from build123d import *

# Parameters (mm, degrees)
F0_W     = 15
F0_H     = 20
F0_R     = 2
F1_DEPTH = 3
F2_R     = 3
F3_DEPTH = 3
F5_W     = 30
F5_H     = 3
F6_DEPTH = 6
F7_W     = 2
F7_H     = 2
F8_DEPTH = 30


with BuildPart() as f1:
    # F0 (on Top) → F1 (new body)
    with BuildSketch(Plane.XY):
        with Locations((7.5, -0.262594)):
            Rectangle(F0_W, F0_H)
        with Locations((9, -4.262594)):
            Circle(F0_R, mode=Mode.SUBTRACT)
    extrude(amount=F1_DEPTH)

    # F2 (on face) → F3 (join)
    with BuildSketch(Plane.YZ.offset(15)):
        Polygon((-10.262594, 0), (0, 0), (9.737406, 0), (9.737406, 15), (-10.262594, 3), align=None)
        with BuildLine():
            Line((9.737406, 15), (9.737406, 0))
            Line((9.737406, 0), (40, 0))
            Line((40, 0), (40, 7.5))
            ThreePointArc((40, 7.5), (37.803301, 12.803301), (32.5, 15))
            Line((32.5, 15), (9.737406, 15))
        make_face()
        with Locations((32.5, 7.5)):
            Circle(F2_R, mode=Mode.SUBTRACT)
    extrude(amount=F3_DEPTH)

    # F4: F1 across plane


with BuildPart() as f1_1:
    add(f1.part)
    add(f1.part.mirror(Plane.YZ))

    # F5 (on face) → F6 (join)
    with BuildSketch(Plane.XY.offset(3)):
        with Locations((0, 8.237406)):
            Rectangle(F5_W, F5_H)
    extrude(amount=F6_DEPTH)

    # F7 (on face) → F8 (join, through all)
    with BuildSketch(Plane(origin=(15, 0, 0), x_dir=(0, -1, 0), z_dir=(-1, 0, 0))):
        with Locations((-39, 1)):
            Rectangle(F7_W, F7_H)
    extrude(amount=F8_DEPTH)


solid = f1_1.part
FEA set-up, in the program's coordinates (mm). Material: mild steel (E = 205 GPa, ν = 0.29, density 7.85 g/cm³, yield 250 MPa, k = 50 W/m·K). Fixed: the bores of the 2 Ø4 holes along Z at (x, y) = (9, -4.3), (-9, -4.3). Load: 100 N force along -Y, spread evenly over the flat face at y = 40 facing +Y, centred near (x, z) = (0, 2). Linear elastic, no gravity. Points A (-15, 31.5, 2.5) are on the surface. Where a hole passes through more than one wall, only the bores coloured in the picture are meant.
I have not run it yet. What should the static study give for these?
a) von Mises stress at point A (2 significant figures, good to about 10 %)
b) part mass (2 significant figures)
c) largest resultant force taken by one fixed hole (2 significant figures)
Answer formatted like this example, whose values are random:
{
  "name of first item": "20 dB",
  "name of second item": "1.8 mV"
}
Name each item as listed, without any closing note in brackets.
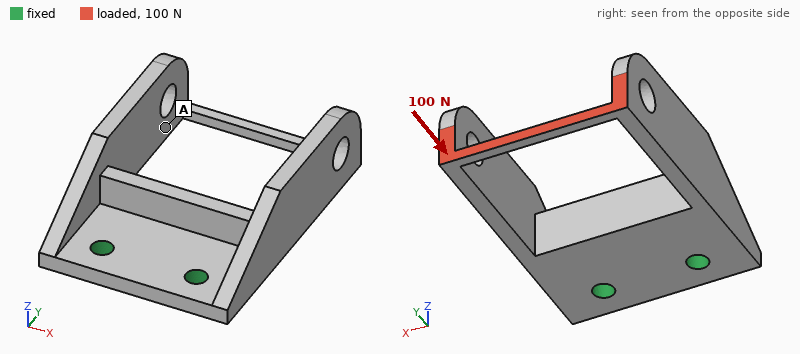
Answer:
{
  "von Mises stress at point A": "13 MPa",
  "part mass": "47 g",
  "largest resultant force taken by one fixed hole": "55 N"
}
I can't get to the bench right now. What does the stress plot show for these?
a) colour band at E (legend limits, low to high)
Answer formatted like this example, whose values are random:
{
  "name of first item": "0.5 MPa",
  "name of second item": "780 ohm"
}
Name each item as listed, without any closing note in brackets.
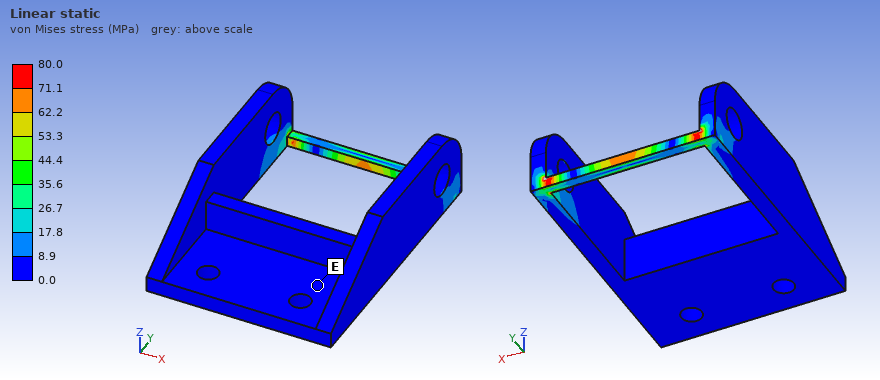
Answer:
{
  "colour band at E": "0.0 to 8.9 MPa"
}
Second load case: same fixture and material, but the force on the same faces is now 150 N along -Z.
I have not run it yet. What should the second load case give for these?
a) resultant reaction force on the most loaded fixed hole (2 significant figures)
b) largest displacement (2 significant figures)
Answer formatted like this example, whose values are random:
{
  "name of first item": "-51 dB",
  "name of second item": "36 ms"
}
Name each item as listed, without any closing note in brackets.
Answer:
{
  "resultant reaction force on the most loaded fixed hole": "81 N",
  "largest displacement": "0.11 mm"
}
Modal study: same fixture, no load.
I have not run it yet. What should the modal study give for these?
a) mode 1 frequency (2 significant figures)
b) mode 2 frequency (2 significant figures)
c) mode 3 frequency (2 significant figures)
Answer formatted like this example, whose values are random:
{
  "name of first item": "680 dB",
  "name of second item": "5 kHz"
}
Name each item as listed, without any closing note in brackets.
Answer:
{
  "mode 1 frequency": "2300 Hz",
  "mode 2 frequency": "2300 Hz",
  "mode 3 frequency": "2500 Hz"
}
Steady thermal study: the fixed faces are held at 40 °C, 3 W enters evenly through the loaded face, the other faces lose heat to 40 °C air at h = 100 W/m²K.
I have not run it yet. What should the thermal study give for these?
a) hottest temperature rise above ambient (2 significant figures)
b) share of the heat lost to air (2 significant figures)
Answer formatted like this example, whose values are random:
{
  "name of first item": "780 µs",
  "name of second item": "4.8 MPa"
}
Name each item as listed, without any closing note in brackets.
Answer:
{
  "hottest temperature rise above ambient": "40 K",
  "share of the heat lost to air": "78 %"
}
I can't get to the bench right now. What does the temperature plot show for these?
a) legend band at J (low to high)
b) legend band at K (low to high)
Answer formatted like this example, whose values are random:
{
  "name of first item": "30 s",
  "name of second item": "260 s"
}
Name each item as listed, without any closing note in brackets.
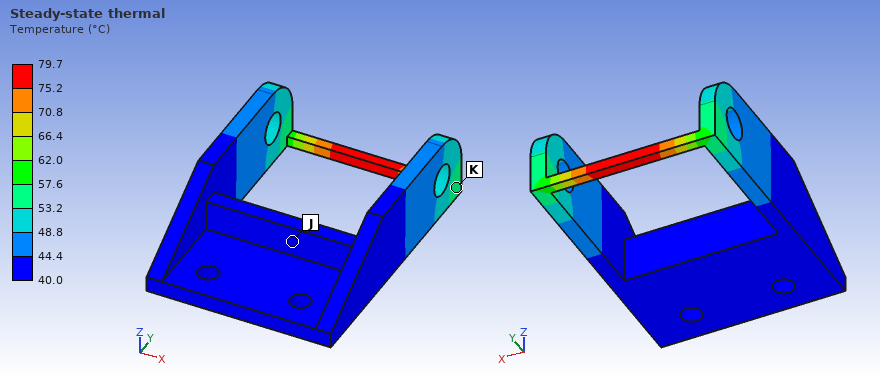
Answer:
{
  "legend band at J": "40.0 to 44.4 °C",
  "legend band at K": "53.2 to 57.6 °C"
}
